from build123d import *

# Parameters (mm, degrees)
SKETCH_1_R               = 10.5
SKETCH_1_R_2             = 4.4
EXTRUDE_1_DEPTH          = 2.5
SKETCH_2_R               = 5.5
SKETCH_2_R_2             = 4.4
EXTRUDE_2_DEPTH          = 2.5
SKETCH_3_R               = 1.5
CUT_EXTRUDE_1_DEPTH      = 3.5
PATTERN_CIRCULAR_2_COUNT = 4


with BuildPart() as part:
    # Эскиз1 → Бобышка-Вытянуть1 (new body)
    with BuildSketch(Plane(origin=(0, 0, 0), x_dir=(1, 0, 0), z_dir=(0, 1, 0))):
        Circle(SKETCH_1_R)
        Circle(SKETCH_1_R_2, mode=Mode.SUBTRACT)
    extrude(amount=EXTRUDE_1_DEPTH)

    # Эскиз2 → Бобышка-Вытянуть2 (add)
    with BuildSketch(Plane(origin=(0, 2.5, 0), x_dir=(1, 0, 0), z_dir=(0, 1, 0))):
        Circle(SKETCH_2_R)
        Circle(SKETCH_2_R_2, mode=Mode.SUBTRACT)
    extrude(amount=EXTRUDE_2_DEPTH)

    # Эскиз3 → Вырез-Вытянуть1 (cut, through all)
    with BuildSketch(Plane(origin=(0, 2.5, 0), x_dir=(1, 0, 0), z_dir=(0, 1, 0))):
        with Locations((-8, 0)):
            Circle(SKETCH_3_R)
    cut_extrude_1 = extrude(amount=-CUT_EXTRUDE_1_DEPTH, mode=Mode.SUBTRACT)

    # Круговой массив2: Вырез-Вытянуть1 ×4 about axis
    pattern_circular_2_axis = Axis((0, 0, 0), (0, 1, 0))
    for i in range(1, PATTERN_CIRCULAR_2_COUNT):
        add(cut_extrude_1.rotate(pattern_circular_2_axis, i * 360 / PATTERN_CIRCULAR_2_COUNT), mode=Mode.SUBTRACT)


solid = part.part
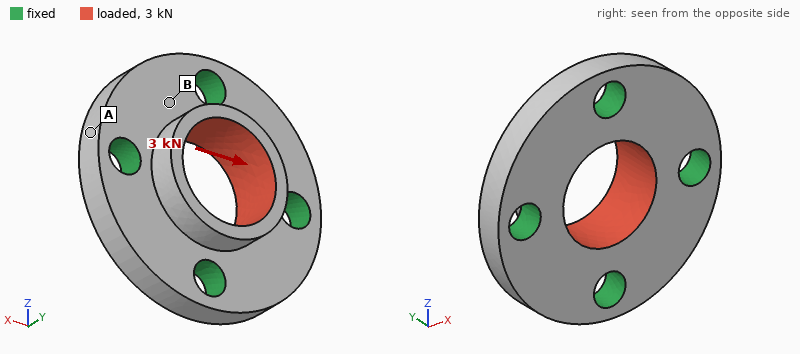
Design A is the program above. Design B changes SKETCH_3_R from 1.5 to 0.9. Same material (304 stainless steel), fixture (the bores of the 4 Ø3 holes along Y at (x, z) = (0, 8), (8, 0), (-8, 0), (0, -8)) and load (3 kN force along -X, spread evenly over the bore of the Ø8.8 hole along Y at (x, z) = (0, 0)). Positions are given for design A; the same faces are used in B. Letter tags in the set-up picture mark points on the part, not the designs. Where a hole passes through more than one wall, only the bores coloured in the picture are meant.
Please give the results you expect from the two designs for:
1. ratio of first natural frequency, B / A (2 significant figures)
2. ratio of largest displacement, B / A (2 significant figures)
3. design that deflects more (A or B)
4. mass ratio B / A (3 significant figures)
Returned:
0.78
1.1
B
1.06
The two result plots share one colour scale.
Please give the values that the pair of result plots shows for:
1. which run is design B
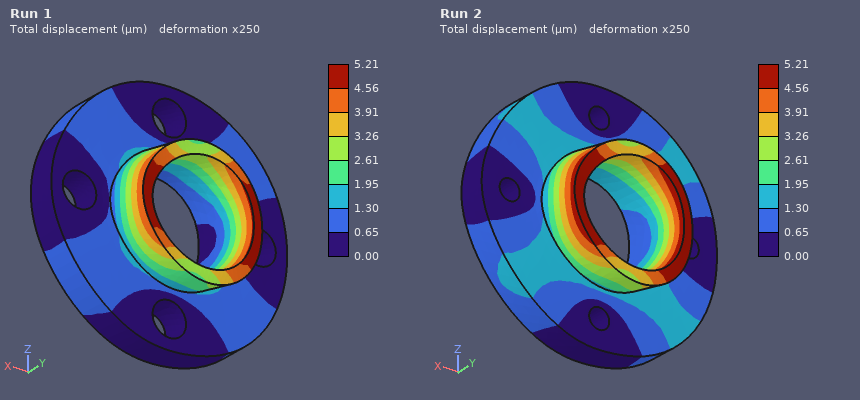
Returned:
Run 2
